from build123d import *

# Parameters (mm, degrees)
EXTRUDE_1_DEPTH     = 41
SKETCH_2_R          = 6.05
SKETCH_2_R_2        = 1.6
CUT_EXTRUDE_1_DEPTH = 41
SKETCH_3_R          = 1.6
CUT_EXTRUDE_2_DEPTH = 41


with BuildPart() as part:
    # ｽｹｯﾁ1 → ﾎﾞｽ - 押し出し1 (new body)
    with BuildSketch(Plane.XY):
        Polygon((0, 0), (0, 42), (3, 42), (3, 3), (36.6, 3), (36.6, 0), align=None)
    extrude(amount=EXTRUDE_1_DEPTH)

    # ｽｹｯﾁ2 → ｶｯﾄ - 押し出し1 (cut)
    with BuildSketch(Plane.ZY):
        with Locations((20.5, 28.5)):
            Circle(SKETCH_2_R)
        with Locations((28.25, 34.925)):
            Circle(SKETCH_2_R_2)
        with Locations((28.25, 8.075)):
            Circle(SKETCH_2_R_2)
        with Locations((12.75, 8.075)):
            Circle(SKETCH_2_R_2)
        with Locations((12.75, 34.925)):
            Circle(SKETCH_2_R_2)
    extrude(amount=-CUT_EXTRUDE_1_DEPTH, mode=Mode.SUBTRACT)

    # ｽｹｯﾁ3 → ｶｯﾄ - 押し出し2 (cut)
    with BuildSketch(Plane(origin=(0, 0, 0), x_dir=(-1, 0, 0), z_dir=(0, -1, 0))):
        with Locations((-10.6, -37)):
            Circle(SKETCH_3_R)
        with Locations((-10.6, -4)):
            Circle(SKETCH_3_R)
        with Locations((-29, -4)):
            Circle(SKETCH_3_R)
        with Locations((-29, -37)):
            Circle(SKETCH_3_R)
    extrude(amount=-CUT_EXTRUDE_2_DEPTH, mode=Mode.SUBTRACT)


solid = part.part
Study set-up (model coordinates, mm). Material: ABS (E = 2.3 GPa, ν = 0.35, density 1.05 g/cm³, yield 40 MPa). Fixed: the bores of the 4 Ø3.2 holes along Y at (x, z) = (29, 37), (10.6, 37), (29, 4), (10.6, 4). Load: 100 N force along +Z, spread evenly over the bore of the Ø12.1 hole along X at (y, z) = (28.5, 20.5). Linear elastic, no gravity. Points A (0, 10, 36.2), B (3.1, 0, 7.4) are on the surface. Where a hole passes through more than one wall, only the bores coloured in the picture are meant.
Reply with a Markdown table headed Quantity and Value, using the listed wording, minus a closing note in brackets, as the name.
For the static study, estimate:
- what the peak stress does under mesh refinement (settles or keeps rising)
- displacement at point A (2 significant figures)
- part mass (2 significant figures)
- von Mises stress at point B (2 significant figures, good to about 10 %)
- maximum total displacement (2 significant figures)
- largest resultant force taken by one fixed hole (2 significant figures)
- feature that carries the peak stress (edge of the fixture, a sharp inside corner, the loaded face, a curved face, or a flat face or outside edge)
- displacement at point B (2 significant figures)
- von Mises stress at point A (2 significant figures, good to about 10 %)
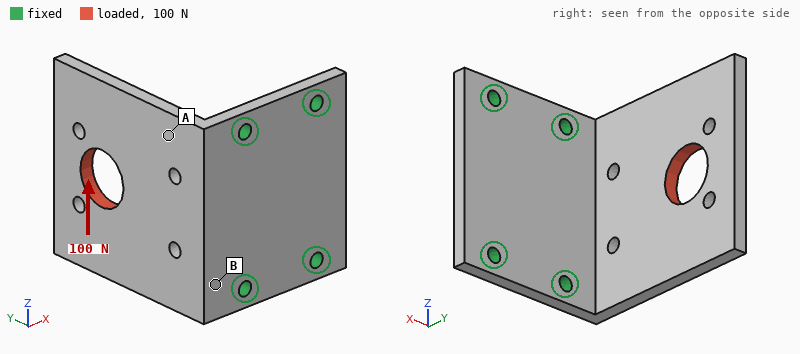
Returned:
| Quantity | Value |
|---|---|
| what the peak stress does under mesh refinement | keeps rising |
| displacement at point A | 0.26 mm |
| part mass | 9.2 g |
| von Mises stress at point B | 7.3 MPa |
| maximum total displacement | 0.69 mm |
| largest resultant force taken by one fixed hole | 100 N |
| feature that carries the peak stress | edge of the fixture |
| displacement at point B | 0.12 mm |
| von Mises stress at point A | 2.6 MPa |
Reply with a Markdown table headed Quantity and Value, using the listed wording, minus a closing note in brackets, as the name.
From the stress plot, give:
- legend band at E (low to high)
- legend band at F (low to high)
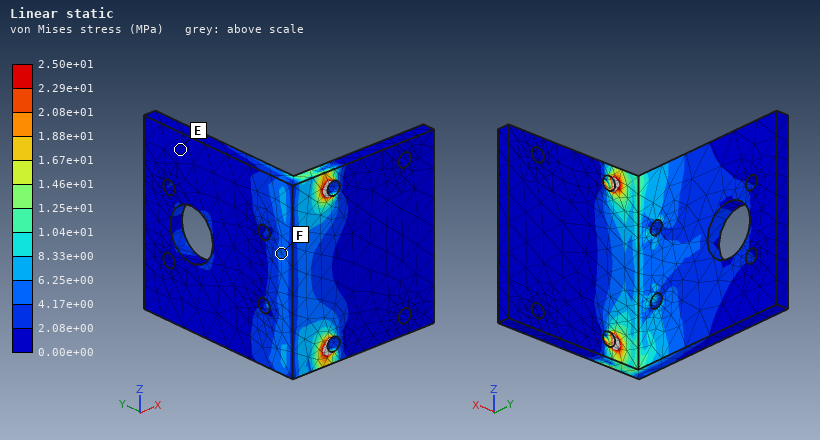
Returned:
| Quantity | Value |
|---|---|
| legend band at E | 0.00e+00 to 2.08e+00 MPa |
| legend band at F | 4.17e+00 to 6.25e+00 MPa |
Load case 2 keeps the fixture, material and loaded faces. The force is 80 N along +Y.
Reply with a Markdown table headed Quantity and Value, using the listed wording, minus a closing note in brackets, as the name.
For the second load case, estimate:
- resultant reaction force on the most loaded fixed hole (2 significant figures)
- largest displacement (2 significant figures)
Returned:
| Quantity | Value |
|---|---|
| resultant reaction force on the most loaded fixed hole | 45 N |
| largest displacement | 0.70 mm |
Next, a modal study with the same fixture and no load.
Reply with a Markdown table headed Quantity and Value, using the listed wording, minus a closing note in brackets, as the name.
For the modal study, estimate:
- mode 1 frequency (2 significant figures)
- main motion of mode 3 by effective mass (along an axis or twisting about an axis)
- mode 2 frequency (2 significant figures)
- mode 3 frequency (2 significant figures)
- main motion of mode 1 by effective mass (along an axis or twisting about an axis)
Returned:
| Quantity | Value |
|---|---|
| mode 1 frequency | 340 Hz |
| main motion of mode 3 by effective mass | along Z |
| mode 2 frequency | 860 Hz |
| mode 3 frequency | 1400 Hz |
| main motion of mode 1 by effective mass | along X |
